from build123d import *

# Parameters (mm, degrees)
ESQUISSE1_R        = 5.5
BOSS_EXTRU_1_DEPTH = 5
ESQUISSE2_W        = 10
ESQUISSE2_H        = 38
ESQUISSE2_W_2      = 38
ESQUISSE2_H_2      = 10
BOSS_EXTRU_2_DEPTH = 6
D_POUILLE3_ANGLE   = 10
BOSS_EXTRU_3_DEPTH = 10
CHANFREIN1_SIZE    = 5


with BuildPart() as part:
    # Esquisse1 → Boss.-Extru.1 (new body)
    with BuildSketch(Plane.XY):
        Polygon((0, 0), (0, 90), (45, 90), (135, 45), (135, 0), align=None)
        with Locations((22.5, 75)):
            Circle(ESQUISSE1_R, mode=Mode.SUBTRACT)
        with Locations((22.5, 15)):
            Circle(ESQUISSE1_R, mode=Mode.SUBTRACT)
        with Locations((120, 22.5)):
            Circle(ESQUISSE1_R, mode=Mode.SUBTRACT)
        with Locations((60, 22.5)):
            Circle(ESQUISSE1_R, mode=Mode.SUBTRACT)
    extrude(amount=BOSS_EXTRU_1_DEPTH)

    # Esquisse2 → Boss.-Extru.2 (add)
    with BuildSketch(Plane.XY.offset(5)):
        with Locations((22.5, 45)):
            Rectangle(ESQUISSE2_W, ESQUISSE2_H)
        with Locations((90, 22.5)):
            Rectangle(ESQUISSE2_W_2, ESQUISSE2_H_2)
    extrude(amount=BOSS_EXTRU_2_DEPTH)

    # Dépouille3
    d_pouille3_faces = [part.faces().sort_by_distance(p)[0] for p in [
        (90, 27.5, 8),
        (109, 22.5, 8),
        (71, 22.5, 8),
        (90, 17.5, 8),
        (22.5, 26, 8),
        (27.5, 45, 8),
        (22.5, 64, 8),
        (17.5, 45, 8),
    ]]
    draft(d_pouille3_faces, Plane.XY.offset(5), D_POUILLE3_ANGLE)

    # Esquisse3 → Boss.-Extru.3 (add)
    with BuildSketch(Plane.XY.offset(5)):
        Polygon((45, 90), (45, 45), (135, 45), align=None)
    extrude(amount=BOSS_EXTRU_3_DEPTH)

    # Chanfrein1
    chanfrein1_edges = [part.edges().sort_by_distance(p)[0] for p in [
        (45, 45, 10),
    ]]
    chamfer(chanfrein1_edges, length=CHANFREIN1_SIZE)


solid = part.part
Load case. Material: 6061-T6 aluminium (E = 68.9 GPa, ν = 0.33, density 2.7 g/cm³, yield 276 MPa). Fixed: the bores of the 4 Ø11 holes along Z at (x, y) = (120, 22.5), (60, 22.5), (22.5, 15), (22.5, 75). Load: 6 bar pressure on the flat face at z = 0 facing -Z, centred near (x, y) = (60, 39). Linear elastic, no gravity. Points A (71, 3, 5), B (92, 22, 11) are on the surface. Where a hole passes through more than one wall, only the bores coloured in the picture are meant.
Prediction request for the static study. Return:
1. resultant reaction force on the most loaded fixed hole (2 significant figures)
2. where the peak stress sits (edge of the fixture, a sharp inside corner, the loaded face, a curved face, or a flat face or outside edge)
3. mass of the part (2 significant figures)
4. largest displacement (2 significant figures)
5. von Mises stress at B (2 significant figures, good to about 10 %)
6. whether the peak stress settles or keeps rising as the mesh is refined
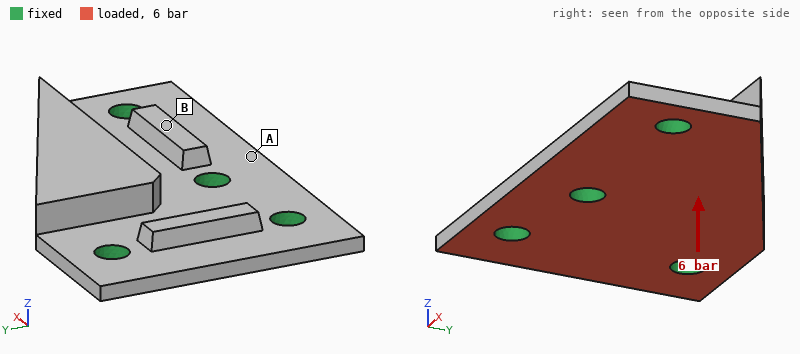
1.9 kN
edge of the fixture
200 g
81 µm
22 MPa
keeps rising
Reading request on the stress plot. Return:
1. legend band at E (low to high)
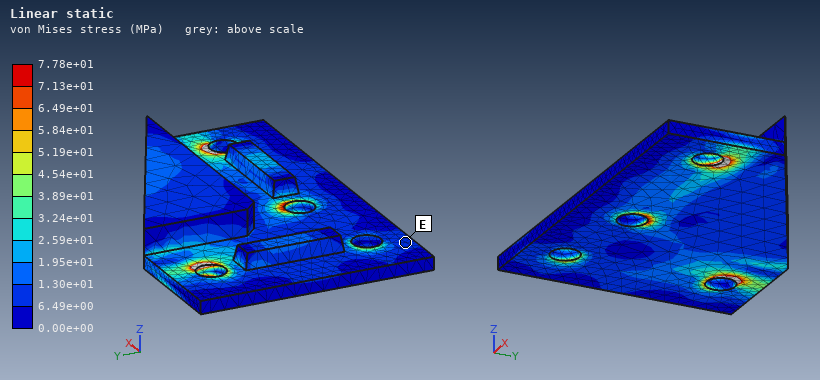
6.49e+00 to 1.30e+01 MPa
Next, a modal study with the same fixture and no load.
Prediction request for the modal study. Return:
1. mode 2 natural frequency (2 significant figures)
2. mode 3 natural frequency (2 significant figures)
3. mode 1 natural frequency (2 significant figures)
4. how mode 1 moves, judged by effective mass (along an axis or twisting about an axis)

6400 Hz
7700 Hz
2800 Hz
along Z
